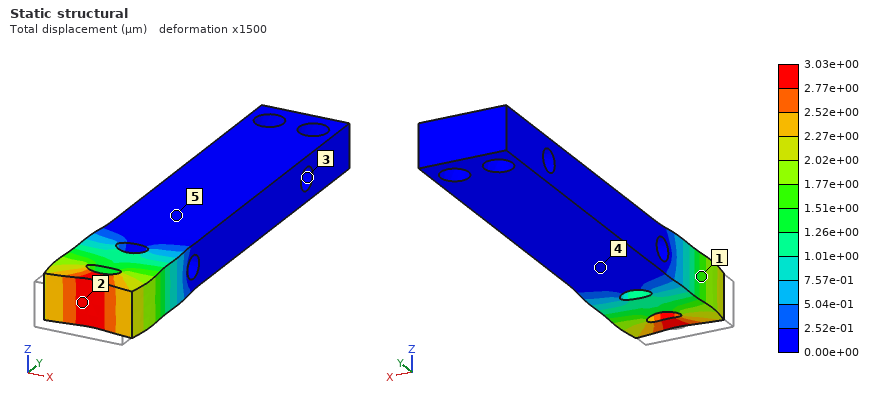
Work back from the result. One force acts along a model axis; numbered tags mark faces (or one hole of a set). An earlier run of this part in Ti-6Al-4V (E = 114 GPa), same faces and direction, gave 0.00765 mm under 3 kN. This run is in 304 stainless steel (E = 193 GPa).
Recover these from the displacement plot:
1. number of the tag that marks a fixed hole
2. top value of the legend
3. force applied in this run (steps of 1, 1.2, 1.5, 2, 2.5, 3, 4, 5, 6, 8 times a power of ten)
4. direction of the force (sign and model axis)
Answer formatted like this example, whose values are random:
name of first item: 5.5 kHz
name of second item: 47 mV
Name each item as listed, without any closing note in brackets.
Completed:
number of the tag that marks a fixed hole: 3
top value of the legend: 3.03e+00 µm
force applied in this run: 2 kN
direction of the force: +Y
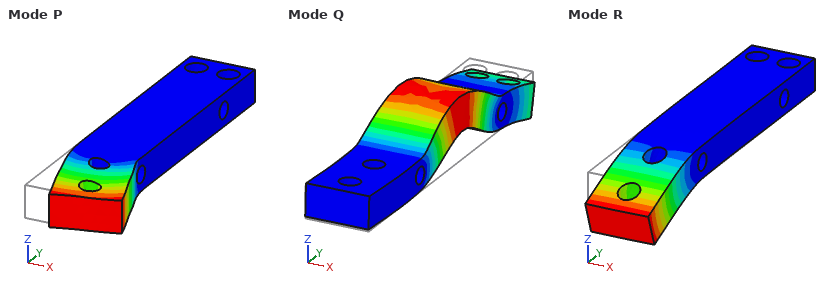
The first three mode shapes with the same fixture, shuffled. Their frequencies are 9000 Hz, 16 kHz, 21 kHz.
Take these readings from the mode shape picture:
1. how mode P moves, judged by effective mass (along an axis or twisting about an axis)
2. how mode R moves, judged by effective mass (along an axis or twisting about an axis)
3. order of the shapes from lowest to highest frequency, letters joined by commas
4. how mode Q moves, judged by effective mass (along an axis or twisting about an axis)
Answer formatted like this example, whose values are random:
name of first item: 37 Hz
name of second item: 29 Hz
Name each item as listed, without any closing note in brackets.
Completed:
how mode P moves, judged by effective mass: along X
how mode R moves, judged by effective mass: along Z
order of the shapes from lowest to highest frequency, letters joined by commas: R, P, Q
how mode Q moves, judged by effective mass: along Z
